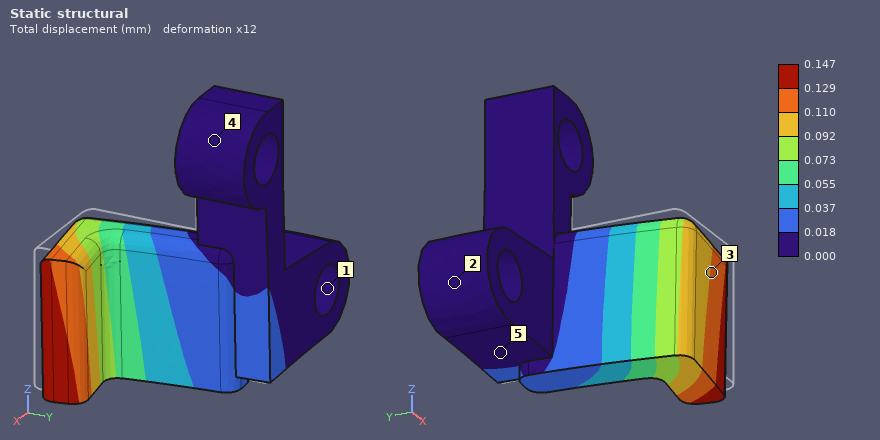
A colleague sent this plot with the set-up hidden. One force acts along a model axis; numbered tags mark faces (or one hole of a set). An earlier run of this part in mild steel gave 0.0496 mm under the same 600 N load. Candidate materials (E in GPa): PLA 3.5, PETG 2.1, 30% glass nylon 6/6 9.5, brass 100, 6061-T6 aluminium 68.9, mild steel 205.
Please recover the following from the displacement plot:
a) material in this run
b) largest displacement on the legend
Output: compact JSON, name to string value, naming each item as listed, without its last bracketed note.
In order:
{"material in this run": "6061-T6 aluminium", "largest displacement on the legend": "0.147 mm"}
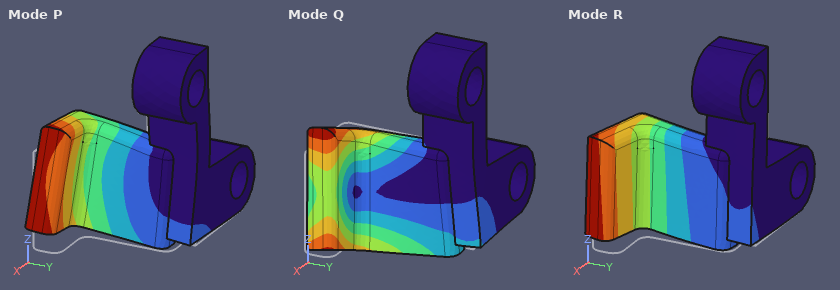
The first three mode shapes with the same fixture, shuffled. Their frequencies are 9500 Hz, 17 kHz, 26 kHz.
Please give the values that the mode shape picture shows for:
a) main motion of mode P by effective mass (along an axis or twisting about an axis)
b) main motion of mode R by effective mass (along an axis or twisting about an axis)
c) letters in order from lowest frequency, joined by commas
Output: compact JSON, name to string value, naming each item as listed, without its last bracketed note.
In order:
{"main motion of mode P by effective mass": "along Z", "main motion of mode R by effective mass": "along X", "letters in order from lowest frequency, joined by commas": "R, P, Q"}
